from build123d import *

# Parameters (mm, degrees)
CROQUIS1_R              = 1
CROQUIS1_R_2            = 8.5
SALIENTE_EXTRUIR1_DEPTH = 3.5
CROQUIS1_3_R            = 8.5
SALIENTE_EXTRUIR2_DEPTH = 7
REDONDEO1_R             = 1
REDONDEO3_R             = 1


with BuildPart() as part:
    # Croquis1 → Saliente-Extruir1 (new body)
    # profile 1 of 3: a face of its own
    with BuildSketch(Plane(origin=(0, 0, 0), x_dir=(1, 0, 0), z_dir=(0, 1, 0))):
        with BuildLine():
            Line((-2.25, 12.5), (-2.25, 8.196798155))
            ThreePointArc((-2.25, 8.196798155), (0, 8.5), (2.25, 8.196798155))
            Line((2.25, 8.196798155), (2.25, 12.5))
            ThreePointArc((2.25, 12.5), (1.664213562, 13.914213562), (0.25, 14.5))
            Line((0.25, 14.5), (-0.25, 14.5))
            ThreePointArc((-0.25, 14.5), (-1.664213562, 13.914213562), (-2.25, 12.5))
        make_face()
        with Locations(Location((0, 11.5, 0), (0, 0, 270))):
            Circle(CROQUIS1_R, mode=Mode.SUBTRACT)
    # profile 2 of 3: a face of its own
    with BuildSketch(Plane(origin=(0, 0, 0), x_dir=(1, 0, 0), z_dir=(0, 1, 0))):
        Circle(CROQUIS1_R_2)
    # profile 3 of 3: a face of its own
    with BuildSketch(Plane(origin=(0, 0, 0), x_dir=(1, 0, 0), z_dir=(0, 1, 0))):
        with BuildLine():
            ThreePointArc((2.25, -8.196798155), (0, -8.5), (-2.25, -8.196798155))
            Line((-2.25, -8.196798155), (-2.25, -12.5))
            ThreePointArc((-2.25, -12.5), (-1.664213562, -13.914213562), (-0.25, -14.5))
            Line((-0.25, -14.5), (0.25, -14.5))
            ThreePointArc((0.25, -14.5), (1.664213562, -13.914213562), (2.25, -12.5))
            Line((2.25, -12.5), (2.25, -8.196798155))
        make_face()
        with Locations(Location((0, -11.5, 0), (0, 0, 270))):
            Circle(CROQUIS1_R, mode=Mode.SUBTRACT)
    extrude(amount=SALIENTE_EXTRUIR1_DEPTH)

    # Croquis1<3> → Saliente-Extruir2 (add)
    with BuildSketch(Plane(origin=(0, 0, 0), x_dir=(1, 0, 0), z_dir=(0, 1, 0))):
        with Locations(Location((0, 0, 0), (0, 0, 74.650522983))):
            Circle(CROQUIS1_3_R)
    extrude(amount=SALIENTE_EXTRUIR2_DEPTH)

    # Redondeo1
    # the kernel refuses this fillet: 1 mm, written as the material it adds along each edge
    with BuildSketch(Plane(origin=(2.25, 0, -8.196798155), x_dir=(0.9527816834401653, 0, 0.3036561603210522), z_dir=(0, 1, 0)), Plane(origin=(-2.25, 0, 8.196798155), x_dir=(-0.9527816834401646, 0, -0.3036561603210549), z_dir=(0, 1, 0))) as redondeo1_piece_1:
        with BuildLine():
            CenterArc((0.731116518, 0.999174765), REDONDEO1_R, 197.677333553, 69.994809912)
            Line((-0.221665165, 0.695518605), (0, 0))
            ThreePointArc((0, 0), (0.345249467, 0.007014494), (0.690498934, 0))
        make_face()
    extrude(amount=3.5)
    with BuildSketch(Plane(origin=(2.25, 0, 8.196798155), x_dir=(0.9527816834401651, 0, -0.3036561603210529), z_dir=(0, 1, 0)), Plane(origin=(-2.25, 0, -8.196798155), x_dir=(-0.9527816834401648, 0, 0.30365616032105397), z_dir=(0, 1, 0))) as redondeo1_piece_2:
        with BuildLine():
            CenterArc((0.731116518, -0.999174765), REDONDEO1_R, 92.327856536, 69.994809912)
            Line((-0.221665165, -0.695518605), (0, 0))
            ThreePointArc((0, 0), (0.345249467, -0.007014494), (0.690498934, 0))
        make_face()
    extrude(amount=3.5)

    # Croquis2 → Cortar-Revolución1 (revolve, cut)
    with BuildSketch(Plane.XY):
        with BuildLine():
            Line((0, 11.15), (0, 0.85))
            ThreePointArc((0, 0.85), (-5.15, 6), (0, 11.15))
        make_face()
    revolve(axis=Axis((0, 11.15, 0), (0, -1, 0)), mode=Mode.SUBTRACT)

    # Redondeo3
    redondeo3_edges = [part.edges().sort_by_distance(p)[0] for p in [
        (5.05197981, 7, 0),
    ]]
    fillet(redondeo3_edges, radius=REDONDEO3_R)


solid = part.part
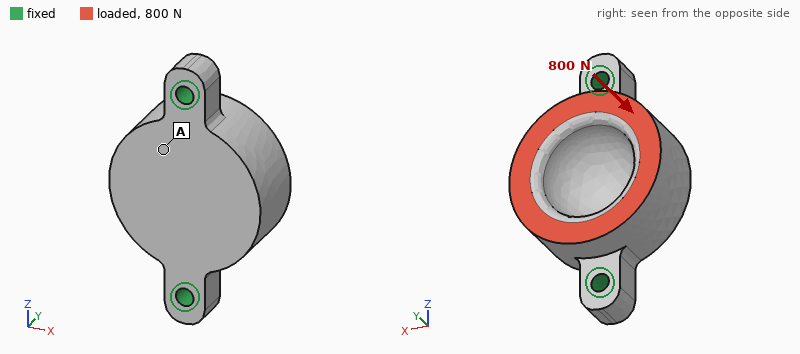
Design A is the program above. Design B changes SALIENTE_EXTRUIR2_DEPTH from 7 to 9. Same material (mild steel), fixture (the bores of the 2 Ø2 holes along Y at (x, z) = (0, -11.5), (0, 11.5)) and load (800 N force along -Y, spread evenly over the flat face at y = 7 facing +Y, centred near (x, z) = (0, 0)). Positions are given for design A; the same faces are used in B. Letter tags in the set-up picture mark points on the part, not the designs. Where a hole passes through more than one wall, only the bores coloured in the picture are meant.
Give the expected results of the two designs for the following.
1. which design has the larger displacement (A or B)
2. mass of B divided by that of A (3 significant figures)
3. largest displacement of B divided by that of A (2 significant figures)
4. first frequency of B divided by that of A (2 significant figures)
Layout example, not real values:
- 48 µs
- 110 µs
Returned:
- A
- 1.22
- 0.74
- 0.80
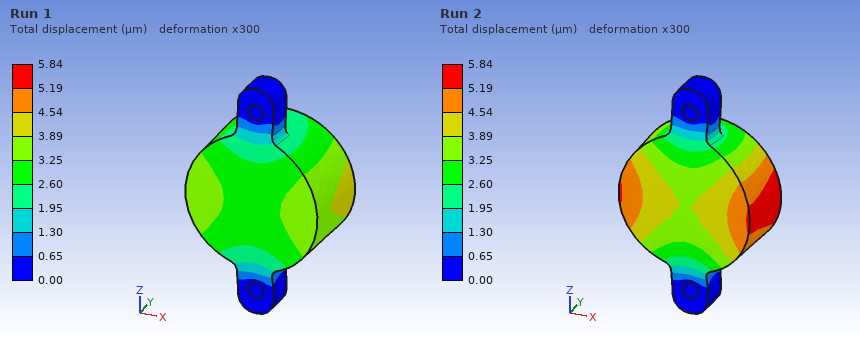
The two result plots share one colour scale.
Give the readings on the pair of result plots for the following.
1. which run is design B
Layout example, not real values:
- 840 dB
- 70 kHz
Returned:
- Run 1
